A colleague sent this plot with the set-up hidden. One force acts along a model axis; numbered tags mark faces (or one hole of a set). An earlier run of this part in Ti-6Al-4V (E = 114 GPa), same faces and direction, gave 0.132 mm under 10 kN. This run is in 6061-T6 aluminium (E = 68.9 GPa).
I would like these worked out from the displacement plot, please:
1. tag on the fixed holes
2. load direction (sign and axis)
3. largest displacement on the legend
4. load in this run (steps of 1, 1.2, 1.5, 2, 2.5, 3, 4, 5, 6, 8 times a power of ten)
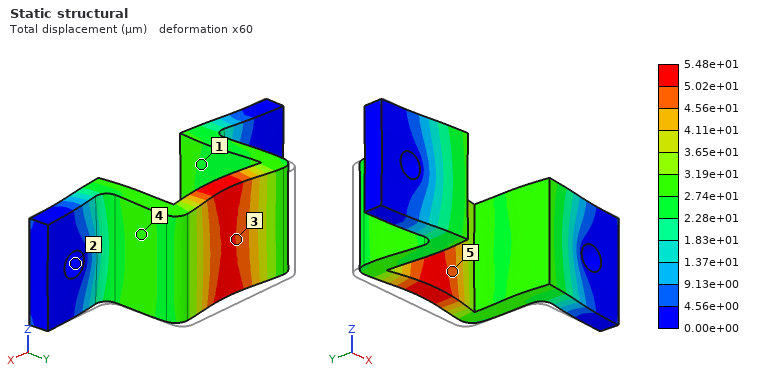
2
-Y
5.48e+01 µm
2.5 kN
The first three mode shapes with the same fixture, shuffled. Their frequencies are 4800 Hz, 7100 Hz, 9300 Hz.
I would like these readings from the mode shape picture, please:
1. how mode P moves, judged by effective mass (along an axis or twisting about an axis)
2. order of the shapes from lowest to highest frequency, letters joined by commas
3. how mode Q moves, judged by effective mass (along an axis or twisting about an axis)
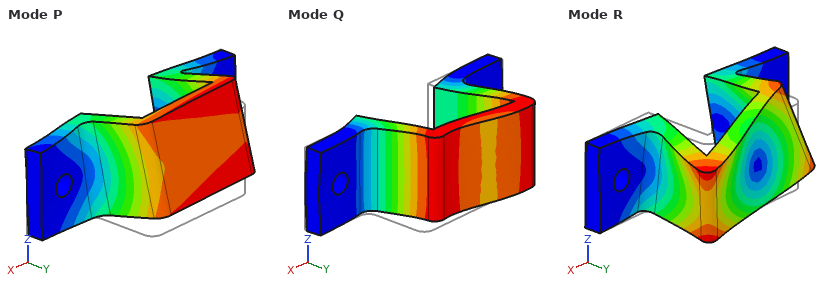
along Z
P, Q, R
along X
